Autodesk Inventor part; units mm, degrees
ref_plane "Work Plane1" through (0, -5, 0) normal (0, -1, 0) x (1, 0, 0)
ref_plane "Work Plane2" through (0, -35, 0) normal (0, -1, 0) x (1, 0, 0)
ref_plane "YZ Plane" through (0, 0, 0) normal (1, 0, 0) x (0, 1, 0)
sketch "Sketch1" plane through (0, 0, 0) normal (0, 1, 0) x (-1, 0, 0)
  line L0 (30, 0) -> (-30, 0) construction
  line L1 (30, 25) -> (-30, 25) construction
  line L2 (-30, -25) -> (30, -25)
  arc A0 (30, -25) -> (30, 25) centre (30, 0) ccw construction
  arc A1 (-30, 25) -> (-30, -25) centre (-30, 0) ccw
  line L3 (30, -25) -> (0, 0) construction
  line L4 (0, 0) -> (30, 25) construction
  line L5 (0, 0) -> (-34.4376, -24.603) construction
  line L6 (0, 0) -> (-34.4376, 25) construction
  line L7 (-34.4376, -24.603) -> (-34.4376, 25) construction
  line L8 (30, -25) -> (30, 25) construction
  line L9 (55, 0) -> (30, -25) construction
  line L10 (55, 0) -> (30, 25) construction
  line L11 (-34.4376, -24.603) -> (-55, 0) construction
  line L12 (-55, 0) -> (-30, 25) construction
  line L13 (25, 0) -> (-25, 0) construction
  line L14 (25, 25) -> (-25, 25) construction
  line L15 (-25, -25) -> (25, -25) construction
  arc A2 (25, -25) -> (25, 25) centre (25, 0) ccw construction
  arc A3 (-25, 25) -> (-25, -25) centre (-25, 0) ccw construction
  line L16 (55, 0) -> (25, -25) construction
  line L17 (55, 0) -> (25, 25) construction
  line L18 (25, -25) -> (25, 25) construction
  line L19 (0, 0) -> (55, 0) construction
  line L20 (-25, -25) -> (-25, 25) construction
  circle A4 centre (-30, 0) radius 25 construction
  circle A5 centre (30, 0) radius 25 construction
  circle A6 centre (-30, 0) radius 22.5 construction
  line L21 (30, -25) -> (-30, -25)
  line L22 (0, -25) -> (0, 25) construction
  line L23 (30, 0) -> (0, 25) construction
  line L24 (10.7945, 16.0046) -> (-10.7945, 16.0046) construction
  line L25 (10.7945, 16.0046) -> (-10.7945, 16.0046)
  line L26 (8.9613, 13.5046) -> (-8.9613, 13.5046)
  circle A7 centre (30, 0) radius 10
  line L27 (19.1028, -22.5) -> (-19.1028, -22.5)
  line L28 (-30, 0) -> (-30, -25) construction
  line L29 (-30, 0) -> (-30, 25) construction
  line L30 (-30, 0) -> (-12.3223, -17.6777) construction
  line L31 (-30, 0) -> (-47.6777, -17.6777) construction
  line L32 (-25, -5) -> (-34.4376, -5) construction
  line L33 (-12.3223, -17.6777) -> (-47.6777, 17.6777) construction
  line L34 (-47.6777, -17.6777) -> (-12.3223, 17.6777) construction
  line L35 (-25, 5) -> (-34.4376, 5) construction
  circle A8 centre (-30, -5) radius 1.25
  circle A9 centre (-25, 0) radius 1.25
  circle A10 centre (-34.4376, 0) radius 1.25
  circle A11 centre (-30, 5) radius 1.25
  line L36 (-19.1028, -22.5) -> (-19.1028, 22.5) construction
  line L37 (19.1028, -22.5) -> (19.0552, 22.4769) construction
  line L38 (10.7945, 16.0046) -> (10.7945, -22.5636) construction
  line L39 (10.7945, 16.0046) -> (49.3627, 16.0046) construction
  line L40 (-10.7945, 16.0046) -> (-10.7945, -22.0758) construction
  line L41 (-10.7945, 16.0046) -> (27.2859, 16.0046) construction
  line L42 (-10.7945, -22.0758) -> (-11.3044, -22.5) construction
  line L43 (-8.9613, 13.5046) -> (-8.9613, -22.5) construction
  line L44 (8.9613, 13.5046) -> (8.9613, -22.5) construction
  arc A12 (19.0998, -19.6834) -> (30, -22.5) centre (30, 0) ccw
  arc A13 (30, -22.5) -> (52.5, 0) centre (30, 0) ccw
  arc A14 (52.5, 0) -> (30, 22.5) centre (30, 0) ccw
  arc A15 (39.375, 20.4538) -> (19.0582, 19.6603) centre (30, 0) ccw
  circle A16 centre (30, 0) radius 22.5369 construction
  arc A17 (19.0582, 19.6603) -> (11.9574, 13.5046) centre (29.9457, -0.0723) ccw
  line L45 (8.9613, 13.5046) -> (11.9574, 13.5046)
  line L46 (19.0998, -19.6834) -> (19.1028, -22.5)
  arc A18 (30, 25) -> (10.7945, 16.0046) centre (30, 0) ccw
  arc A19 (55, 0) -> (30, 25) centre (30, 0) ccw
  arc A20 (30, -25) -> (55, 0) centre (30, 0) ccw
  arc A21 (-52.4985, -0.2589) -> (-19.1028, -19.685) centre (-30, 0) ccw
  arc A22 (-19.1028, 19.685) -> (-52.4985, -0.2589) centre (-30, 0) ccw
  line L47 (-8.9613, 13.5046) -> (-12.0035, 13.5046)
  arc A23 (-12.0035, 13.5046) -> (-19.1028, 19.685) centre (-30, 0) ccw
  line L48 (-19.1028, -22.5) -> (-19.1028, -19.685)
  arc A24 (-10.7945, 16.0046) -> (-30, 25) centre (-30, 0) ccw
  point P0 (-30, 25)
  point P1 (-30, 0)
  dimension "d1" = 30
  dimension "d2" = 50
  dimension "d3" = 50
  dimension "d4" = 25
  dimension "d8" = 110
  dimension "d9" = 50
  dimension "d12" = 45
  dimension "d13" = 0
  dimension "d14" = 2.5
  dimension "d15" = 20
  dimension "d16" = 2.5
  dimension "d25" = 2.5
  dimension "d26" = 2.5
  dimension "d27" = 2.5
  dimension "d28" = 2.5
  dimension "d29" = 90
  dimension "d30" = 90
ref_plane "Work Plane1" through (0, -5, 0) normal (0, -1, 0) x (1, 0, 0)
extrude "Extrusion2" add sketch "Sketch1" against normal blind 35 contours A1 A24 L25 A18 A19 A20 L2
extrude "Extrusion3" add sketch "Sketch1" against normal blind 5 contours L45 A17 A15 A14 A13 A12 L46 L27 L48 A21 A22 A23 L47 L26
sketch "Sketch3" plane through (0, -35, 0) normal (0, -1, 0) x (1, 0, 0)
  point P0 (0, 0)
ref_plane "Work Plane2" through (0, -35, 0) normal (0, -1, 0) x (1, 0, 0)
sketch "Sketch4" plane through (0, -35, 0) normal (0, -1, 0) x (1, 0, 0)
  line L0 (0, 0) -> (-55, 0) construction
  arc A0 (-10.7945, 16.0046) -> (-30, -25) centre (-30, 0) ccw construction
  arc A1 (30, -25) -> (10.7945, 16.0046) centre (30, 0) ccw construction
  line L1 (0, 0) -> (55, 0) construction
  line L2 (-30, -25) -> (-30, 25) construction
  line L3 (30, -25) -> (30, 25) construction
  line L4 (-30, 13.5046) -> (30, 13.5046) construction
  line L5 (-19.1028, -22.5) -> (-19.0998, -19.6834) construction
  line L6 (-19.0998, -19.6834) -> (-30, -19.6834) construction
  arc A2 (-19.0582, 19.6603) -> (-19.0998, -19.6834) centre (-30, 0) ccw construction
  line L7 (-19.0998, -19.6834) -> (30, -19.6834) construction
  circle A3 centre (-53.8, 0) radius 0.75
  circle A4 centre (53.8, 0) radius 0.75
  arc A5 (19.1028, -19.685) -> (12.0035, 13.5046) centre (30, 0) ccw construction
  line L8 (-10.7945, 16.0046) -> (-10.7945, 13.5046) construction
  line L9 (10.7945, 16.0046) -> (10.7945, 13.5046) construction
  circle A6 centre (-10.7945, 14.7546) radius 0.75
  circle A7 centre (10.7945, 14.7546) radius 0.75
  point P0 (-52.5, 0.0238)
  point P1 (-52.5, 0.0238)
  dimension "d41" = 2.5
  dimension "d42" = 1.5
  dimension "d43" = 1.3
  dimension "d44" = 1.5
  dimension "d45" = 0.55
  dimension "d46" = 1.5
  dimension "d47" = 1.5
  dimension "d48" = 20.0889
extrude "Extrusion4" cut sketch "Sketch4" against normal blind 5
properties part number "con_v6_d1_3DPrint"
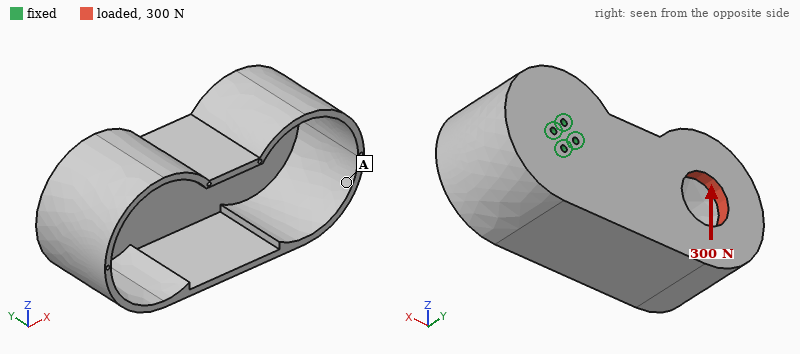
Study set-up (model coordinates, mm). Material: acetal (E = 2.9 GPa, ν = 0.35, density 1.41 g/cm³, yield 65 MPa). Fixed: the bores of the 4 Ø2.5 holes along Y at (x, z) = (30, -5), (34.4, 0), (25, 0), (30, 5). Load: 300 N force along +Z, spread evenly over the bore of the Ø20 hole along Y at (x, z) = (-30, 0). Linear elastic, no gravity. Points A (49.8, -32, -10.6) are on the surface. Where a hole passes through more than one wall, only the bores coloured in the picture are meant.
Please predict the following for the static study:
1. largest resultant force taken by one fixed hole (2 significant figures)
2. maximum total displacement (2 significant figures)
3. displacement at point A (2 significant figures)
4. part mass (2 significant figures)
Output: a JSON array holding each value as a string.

["870 N", "1.2 mm", "0.18 mm", "60 g"]
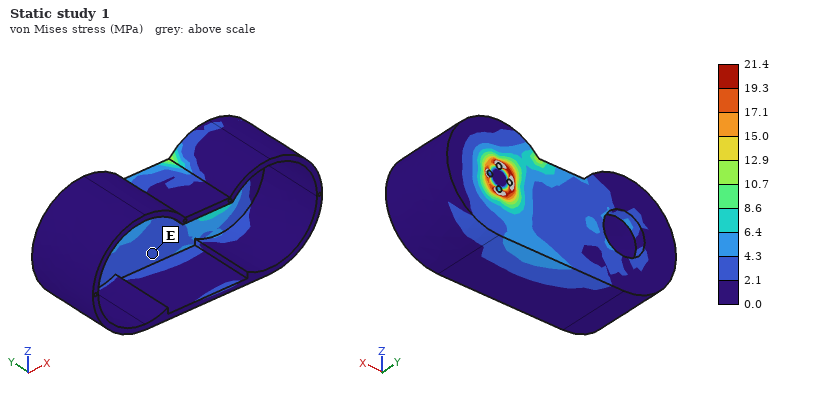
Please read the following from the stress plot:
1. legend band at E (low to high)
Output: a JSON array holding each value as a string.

["2.1 to 4.3 MPa"]
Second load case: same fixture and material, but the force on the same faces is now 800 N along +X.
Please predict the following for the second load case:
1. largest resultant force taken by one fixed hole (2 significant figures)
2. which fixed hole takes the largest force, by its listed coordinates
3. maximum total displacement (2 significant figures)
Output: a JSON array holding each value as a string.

["260 N", "(25, 0)", "0.20 mm"]
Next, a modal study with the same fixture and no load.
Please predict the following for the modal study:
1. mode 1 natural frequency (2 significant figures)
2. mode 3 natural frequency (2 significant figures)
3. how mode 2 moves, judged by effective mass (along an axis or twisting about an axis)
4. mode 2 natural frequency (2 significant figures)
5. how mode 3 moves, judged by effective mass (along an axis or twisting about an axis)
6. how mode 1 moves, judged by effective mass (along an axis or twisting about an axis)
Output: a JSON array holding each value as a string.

["230 Hz", "600 Hz", "along Z", "310 Hz", "along Z", "along Y"]
